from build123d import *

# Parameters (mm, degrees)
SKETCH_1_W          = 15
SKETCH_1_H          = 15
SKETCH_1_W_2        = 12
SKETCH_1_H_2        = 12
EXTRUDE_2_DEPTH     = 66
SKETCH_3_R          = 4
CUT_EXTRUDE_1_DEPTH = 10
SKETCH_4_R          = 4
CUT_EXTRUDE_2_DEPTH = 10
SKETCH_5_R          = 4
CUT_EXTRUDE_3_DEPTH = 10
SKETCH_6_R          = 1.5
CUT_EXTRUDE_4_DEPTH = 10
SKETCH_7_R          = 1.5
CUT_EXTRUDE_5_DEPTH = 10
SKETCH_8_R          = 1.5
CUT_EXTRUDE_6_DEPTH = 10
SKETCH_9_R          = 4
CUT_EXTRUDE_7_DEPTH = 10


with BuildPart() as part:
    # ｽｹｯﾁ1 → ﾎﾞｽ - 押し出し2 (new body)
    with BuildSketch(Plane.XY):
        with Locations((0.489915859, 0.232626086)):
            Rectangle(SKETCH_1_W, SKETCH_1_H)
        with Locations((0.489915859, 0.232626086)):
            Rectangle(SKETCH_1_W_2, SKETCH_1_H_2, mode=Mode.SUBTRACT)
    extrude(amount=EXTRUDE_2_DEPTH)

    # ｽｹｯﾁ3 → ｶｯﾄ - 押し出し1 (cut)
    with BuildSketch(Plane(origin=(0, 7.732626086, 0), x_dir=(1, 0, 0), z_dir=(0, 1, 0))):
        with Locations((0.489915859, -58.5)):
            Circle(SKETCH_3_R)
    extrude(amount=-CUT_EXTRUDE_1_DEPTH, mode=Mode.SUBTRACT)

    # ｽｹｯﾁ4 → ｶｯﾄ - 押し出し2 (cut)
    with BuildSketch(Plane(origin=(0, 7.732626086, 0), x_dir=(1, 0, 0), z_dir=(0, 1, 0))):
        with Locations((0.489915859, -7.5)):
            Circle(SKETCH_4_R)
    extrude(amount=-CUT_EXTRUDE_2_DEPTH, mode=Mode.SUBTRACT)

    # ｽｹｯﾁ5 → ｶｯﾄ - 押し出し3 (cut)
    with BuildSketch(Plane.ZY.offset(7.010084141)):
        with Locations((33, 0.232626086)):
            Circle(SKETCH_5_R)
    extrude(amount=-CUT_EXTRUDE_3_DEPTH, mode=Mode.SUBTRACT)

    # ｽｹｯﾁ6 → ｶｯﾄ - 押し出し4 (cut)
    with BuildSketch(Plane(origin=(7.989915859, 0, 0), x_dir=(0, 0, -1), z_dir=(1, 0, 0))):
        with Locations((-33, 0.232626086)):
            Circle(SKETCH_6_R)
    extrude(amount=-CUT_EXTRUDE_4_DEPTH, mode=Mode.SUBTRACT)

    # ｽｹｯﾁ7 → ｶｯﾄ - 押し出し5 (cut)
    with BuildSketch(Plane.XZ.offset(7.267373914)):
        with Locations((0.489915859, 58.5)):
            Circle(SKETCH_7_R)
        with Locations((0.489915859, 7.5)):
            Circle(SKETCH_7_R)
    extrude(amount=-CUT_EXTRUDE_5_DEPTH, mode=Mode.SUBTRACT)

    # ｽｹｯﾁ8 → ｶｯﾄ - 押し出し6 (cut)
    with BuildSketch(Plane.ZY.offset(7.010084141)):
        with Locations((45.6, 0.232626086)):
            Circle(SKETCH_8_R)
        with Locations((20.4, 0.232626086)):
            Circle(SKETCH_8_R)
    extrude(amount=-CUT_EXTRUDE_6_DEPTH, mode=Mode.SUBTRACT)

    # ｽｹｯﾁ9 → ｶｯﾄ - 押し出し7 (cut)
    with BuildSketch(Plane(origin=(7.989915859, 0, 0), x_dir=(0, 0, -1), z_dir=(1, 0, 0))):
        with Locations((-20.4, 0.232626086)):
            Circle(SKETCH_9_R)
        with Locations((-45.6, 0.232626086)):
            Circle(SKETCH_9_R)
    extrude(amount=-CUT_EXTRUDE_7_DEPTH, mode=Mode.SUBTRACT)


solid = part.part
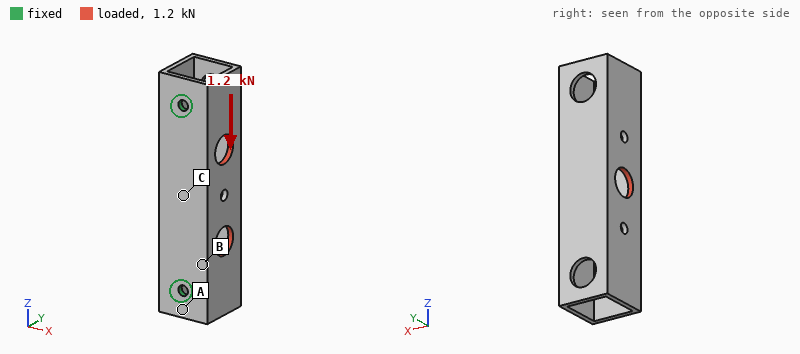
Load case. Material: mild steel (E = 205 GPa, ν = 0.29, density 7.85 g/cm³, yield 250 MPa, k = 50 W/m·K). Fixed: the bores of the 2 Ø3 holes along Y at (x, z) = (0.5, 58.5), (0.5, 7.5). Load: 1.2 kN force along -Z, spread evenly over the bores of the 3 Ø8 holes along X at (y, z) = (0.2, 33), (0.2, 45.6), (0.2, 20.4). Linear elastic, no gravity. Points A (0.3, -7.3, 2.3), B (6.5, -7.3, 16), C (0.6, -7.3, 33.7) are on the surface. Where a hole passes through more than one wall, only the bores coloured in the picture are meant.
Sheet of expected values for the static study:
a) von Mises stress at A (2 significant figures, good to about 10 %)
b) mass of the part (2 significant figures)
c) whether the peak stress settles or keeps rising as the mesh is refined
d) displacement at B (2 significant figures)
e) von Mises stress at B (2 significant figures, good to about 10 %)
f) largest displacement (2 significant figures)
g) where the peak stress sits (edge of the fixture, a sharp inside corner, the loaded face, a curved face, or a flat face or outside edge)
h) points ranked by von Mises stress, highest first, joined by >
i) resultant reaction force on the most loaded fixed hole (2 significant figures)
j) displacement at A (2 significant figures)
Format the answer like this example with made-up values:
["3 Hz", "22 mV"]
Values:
["47 MPa", "39 g", "keeps rising", "2.3 µm", "21 MPa", "8.9 µm", "edge of the fixture", "A > B > C", "620 N", "1.6 µm"]
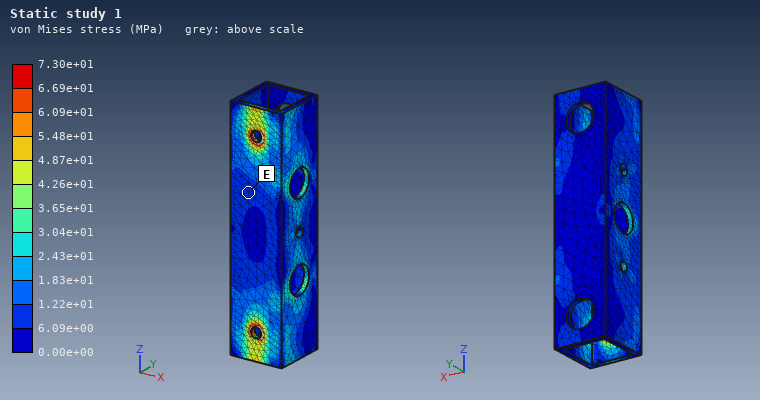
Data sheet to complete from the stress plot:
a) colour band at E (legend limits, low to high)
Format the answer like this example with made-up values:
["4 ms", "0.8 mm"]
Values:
["6.09e+00 to 1.22e+01 MPa"]
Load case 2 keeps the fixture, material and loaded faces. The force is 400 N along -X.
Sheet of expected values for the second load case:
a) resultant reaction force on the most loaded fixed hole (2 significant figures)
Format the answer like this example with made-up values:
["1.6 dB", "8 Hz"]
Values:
["200 N"]
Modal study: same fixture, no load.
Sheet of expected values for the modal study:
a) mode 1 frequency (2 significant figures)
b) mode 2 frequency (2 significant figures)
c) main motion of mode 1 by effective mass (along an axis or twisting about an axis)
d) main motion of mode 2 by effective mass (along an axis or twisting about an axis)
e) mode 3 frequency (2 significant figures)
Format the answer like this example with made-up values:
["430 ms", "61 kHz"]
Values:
["2500 Hz", "6900 Hz", "along X", "along Y", "8900 Hz"]
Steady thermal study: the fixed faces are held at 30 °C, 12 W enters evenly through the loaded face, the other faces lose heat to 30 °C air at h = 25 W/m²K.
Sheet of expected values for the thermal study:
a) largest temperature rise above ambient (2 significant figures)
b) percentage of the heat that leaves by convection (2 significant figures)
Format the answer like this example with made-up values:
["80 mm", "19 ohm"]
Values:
["41 K", "35 %"]
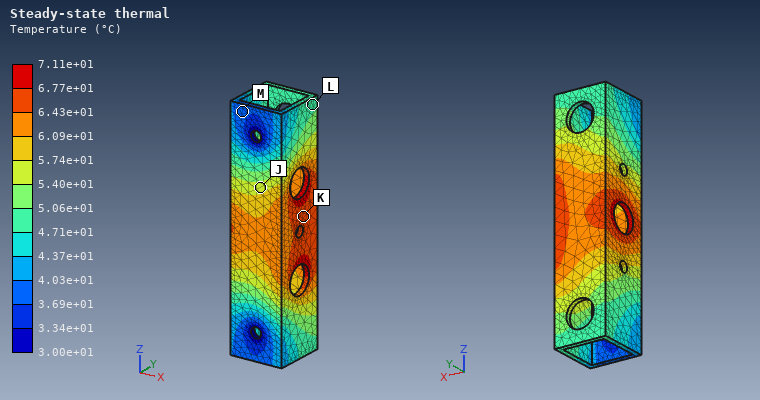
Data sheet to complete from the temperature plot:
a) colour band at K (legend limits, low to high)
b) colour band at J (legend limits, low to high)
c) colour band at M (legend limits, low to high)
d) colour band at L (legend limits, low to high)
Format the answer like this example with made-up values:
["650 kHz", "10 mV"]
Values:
["6.43e+01 to 6.77e+01 °C", "5.40e+01 to 5.74e+01 °C", "3.69e+01 to 4.03e+01 °C", "4.71e+01 to 5.06e+01 °C"]
